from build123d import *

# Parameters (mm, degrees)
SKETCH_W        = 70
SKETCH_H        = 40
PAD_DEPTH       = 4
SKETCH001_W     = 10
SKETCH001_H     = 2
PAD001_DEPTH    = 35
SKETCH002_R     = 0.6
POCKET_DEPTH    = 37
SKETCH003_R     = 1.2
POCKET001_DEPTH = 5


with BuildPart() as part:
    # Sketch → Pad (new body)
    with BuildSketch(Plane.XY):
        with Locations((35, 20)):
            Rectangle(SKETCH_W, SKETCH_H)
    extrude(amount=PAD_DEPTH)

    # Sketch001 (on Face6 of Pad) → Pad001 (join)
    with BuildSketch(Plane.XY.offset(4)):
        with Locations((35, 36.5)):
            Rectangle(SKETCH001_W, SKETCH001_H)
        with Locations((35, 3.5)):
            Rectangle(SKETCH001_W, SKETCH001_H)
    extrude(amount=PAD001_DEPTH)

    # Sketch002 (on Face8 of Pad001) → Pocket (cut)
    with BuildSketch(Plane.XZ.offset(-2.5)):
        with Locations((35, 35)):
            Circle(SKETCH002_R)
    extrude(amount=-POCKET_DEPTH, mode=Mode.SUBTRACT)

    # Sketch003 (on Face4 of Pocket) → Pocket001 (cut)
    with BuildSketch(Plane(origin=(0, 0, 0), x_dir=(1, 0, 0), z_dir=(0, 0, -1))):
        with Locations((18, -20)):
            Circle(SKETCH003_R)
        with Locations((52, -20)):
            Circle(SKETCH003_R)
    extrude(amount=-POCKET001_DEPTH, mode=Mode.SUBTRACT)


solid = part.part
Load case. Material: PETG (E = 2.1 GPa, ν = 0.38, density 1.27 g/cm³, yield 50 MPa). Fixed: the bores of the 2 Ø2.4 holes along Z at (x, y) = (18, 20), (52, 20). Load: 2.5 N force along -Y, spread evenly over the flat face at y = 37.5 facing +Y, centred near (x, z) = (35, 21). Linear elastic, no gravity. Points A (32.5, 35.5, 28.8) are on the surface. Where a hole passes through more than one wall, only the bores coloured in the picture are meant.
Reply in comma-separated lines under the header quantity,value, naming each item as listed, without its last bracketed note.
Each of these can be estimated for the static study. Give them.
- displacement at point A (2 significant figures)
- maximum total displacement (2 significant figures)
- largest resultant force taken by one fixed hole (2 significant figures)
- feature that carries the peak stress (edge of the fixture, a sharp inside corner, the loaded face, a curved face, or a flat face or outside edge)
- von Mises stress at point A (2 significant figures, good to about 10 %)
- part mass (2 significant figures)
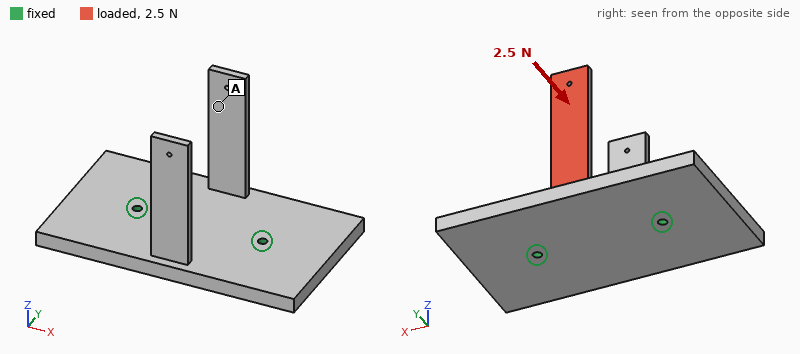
quantity,value
displacement at point A,0.66 mm
maximum total displacement,1.1 mm
largest resultant force taken by one fixed hole,1.3 N
feature that carries the peak stress,the loaded face
von Mises stress at point A,0.57 MPa
part mass,16 g
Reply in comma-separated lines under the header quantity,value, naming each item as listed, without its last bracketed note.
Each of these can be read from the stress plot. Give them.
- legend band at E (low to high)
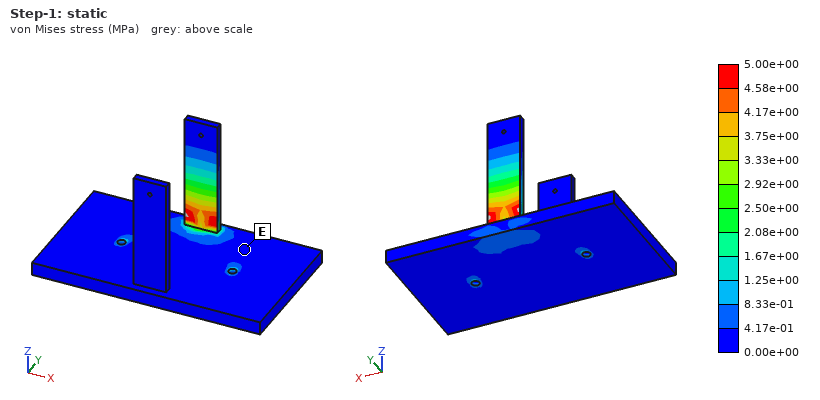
quantity,value
legend band at E,0.00e+00 to 4.17e-01 MPa
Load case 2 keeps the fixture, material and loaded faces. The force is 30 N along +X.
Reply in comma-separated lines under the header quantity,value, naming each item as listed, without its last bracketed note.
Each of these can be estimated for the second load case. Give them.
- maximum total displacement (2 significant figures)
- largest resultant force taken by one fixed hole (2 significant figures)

quantity,value
maximum total displacement,1.0 mm
largest resultant force taken by one fixed hole,28 N
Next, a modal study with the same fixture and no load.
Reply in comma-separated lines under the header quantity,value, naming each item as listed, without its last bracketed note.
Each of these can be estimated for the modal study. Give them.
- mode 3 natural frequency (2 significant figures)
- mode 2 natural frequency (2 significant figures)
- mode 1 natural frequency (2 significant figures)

quantity,value
mode 3 natural frequency,1000 Hz
mode 2 natural frequency,330 Hz
mode 1 natural frequency,320 Hz
